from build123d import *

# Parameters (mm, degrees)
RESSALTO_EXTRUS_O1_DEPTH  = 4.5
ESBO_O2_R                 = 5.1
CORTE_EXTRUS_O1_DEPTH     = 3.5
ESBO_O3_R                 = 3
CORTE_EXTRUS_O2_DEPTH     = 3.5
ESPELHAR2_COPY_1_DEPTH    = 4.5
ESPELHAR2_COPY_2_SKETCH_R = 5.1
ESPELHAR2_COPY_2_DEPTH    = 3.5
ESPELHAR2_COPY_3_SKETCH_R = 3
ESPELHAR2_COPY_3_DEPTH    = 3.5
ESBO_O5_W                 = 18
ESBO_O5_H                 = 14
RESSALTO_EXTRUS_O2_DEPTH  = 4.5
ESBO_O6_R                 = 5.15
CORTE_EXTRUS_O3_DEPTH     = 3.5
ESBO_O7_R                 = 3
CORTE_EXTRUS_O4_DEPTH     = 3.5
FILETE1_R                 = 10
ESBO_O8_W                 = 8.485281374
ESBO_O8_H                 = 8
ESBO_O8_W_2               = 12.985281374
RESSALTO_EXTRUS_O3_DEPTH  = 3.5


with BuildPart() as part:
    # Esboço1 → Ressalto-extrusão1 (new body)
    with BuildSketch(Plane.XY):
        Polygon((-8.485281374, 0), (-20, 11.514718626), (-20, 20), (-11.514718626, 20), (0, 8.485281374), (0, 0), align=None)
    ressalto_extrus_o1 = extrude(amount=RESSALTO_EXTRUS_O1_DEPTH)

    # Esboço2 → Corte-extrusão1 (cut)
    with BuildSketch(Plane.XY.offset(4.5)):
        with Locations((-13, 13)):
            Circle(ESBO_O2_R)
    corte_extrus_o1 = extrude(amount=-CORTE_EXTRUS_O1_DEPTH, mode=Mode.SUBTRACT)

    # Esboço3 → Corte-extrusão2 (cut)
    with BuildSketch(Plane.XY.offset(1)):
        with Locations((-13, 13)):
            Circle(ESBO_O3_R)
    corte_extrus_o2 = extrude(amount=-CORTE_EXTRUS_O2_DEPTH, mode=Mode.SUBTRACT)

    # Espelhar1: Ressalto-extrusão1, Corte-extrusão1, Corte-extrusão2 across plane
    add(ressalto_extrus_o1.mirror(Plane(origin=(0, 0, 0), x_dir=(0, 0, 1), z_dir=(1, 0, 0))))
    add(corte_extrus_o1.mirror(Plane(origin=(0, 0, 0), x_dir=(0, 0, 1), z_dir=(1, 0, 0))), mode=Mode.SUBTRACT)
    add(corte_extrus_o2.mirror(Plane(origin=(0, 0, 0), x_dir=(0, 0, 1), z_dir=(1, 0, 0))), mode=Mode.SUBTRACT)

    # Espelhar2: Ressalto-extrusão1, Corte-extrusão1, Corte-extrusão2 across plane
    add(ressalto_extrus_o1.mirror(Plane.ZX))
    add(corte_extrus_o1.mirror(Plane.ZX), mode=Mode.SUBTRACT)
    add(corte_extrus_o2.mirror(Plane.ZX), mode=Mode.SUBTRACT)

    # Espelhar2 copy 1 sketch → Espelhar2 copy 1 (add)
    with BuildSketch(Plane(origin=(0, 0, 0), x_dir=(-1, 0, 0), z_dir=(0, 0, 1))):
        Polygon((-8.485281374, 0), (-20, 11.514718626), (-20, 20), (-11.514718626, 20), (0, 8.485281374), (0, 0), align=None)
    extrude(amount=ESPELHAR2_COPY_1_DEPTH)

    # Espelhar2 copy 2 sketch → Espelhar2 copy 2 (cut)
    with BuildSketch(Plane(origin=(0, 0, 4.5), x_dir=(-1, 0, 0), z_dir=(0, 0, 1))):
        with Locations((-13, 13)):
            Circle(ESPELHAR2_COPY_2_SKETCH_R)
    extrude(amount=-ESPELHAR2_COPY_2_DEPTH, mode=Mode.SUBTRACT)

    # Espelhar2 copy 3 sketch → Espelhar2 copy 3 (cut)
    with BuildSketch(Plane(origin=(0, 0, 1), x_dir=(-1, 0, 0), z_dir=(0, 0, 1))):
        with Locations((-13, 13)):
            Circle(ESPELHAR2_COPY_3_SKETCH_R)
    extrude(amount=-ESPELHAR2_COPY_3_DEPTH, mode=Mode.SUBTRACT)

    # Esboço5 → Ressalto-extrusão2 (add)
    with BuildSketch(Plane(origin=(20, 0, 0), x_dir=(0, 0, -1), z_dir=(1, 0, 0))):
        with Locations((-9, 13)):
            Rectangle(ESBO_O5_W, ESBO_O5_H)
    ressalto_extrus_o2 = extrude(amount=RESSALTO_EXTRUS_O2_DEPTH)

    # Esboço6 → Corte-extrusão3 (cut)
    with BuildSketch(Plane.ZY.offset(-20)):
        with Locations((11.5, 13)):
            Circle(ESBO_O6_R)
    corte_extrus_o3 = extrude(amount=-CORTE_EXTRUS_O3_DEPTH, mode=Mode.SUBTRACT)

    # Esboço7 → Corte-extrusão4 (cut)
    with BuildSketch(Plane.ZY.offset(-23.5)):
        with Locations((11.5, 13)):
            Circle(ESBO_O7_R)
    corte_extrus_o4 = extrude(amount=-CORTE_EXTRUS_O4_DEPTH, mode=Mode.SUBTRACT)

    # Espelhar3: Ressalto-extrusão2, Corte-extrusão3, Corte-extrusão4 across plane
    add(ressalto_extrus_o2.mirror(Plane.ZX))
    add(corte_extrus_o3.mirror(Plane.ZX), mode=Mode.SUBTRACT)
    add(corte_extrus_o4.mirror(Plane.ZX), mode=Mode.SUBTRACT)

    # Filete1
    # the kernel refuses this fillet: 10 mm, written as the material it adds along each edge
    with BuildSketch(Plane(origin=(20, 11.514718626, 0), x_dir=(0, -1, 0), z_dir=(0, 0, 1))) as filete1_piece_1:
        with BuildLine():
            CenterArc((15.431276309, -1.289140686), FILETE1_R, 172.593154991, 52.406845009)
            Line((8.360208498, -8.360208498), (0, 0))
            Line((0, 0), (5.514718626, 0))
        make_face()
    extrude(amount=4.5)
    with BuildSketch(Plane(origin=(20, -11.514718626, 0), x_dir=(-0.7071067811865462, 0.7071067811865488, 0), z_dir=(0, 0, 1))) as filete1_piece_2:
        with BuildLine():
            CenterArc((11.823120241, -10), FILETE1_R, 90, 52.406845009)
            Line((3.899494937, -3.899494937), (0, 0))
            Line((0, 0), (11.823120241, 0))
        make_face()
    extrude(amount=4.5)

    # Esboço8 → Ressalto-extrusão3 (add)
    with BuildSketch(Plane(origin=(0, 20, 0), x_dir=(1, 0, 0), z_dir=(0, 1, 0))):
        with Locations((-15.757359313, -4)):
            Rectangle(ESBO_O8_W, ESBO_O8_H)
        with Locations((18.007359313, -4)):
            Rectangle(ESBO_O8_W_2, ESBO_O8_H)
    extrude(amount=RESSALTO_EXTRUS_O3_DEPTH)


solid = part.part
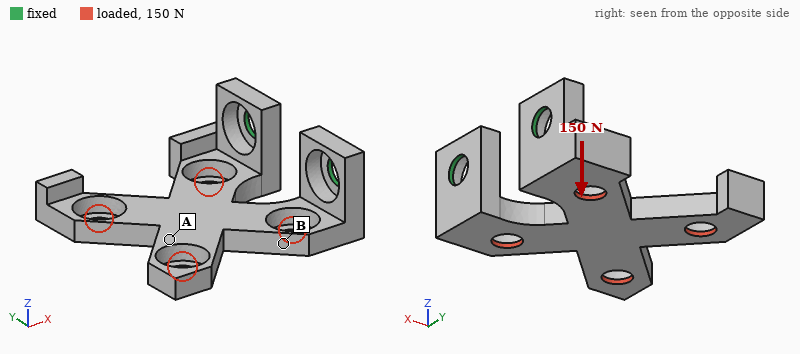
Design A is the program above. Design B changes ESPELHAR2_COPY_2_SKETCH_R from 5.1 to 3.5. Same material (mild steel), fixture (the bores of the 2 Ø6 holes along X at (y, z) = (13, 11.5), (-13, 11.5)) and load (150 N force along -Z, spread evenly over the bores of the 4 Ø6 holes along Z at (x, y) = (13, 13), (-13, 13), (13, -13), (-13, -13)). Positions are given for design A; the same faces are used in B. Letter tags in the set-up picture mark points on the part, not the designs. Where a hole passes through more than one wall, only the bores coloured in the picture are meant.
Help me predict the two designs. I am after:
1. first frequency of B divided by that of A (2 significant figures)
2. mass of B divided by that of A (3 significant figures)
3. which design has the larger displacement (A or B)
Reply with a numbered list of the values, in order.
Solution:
1. 1.0
2. 1.03
3. A
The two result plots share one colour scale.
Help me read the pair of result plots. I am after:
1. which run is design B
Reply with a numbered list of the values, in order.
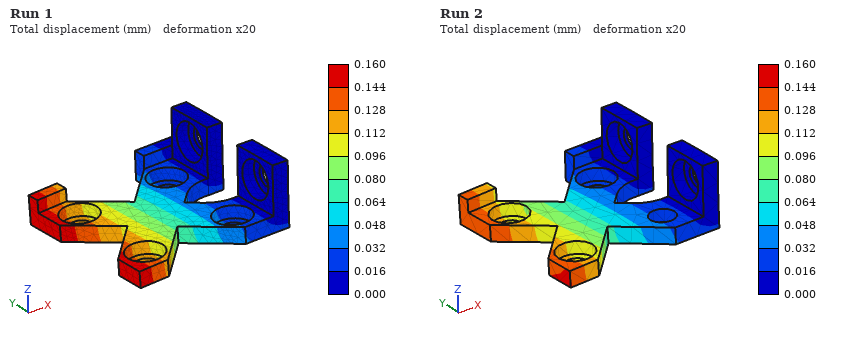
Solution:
1. Run 2
